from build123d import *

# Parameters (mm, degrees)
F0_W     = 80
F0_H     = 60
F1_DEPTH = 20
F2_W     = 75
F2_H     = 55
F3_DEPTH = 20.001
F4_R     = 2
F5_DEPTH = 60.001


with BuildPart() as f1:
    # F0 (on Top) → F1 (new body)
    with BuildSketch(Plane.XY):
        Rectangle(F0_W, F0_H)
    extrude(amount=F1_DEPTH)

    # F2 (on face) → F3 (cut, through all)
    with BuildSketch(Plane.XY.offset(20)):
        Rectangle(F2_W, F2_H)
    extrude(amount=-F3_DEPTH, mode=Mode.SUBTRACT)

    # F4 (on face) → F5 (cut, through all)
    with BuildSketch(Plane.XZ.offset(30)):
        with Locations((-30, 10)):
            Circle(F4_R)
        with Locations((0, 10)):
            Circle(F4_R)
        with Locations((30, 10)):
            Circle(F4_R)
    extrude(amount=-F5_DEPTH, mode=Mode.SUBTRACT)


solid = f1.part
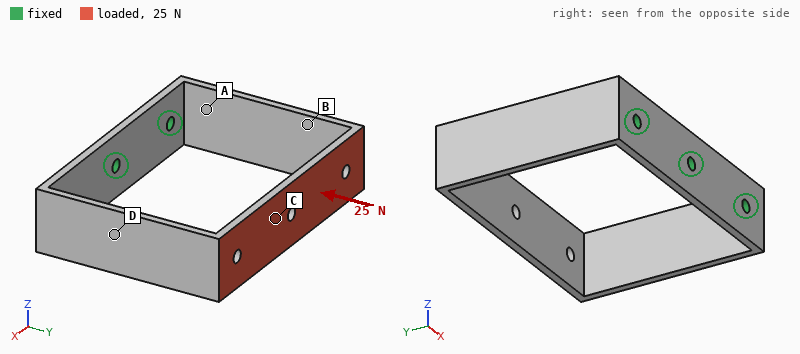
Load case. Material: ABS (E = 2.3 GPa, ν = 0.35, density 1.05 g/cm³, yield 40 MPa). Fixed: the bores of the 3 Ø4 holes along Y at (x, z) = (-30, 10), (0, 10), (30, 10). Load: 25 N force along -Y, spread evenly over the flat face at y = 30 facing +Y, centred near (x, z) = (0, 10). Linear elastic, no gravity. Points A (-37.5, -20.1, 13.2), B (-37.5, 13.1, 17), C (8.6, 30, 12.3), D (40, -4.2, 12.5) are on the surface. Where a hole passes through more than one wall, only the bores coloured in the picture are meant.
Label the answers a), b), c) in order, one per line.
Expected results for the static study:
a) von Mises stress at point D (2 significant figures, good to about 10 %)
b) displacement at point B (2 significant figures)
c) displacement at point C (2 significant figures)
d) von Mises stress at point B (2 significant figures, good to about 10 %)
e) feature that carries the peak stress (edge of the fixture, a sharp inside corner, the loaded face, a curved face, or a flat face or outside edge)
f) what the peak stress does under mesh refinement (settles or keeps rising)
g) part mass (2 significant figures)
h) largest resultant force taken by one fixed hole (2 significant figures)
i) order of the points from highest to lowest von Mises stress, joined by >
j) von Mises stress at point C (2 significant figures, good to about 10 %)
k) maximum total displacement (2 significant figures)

a) 1.4 MPa
b) 0.30 mm
c) 1.1 mm
d) 3.8 MPa
e) edge of the fixture
f) keeps rising
g) 14 g
h) 13 N
i) C > B > D > A
j) 5.1 MPa
k) 1.2 mm
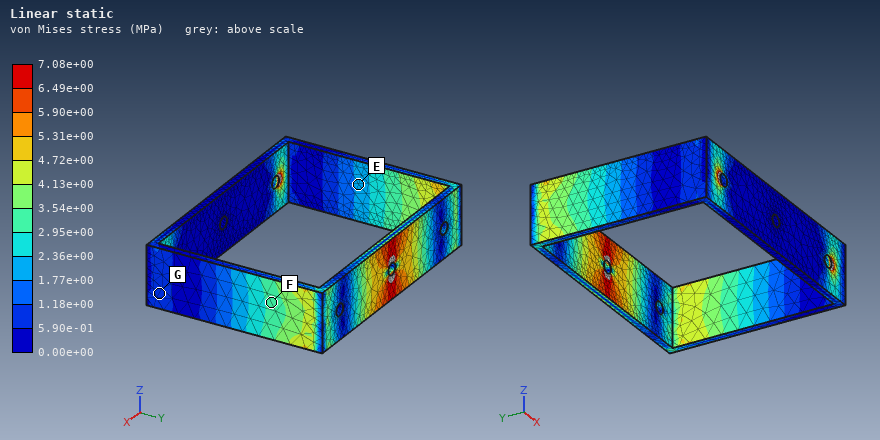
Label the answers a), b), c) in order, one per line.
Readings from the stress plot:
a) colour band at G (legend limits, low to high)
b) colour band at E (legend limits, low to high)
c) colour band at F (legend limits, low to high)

a) 5.90e-01 to 1.18e+00 MPa
b) 1.77e+00 to 2.36e+00 MPa
c) 2.95e+00 to 3.54e+00 MPa
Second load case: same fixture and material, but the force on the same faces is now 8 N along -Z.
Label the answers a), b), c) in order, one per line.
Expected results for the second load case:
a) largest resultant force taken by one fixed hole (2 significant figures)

a) 5.0 N
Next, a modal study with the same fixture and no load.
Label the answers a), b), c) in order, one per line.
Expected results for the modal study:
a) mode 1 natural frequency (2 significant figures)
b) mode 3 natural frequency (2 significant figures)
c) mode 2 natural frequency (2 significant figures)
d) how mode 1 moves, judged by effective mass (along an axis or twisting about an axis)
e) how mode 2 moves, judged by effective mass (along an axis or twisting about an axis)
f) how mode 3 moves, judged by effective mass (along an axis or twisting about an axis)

a) 120 Hz
b) 310 Hz
c) 190 Hz
d) along X
e) along Z
f) twisting about Y
